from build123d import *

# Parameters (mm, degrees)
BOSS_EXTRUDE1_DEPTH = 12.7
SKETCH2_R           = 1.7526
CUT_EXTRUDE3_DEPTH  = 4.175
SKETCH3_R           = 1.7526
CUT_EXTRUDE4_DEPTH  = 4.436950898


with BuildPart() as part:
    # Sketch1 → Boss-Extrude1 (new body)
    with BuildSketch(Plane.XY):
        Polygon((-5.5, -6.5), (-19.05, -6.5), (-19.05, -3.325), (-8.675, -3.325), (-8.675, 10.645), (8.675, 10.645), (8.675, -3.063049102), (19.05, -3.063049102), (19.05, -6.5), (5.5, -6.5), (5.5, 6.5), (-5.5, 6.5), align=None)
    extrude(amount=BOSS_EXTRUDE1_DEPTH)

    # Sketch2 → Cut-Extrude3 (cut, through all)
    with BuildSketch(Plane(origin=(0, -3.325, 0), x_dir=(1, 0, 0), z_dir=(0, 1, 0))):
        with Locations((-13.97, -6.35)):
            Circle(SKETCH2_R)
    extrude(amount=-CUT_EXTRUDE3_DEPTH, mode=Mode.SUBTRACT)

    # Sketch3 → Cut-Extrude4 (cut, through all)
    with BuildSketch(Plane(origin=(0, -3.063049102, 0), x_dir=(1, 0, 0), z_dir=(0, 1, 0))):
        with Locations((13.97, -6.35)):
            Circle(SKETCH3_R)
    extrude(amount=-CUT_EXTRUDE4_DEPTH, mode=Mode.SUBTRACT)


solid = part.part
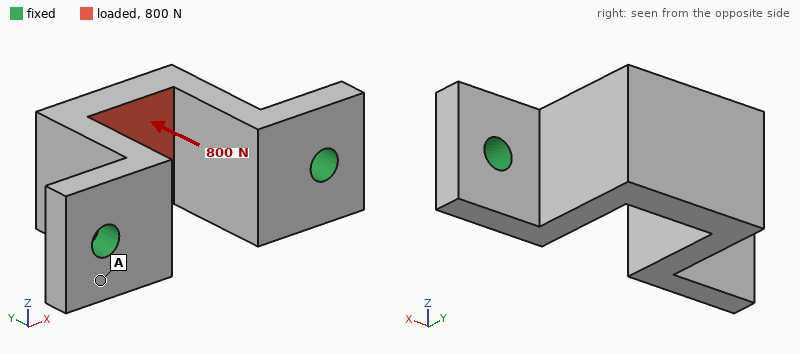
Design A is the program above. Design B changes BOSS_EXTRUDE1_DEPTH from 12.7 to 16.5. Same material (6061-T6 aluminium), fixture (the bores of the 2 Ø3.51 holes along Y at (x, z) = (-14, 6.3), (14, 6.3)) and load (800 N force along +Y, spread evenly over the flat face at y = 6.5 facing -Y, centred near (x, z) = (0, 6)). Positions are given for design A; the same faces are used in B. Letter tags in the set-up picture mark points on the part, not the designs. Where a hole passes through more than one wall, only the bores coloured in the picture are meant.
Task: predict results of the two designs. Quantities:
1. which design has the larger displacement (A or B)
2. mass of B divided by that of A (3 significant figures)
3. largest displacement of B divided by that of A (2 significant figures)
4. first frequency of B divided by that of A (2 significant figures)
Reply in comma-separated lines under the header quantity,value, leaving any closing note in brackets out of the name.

quantity,value
which design has the larger displacement,B
mass of B divided by that of A,1.31
largest displacement of B divided by that of A,1.7
first frequency of B divided by that of A,0.91
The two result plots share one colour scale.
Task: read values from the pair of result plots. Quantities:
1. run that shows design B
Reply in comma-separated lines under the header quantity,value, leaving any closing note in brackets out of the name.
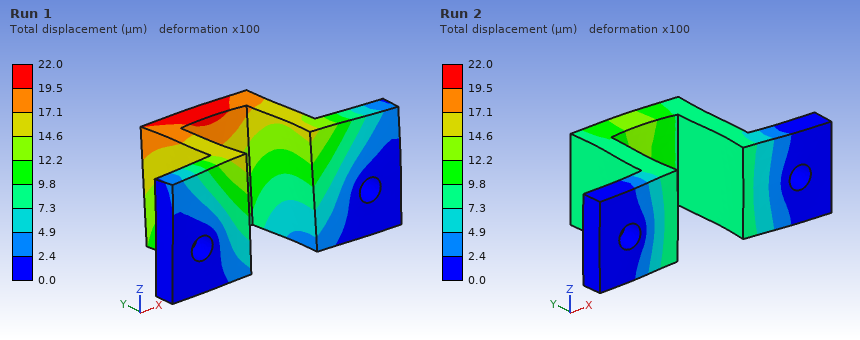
quantity,value
run that shows design B,Run 1
